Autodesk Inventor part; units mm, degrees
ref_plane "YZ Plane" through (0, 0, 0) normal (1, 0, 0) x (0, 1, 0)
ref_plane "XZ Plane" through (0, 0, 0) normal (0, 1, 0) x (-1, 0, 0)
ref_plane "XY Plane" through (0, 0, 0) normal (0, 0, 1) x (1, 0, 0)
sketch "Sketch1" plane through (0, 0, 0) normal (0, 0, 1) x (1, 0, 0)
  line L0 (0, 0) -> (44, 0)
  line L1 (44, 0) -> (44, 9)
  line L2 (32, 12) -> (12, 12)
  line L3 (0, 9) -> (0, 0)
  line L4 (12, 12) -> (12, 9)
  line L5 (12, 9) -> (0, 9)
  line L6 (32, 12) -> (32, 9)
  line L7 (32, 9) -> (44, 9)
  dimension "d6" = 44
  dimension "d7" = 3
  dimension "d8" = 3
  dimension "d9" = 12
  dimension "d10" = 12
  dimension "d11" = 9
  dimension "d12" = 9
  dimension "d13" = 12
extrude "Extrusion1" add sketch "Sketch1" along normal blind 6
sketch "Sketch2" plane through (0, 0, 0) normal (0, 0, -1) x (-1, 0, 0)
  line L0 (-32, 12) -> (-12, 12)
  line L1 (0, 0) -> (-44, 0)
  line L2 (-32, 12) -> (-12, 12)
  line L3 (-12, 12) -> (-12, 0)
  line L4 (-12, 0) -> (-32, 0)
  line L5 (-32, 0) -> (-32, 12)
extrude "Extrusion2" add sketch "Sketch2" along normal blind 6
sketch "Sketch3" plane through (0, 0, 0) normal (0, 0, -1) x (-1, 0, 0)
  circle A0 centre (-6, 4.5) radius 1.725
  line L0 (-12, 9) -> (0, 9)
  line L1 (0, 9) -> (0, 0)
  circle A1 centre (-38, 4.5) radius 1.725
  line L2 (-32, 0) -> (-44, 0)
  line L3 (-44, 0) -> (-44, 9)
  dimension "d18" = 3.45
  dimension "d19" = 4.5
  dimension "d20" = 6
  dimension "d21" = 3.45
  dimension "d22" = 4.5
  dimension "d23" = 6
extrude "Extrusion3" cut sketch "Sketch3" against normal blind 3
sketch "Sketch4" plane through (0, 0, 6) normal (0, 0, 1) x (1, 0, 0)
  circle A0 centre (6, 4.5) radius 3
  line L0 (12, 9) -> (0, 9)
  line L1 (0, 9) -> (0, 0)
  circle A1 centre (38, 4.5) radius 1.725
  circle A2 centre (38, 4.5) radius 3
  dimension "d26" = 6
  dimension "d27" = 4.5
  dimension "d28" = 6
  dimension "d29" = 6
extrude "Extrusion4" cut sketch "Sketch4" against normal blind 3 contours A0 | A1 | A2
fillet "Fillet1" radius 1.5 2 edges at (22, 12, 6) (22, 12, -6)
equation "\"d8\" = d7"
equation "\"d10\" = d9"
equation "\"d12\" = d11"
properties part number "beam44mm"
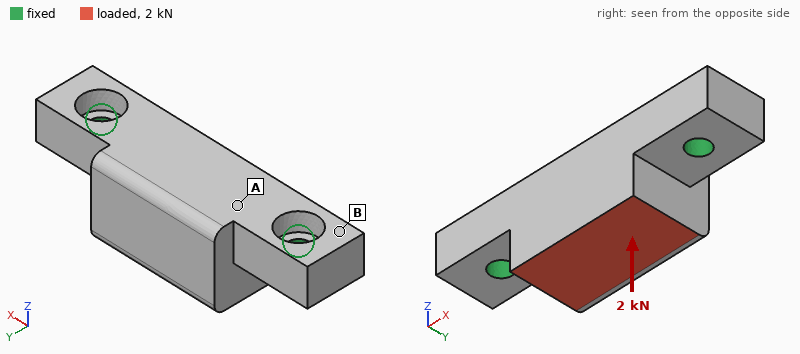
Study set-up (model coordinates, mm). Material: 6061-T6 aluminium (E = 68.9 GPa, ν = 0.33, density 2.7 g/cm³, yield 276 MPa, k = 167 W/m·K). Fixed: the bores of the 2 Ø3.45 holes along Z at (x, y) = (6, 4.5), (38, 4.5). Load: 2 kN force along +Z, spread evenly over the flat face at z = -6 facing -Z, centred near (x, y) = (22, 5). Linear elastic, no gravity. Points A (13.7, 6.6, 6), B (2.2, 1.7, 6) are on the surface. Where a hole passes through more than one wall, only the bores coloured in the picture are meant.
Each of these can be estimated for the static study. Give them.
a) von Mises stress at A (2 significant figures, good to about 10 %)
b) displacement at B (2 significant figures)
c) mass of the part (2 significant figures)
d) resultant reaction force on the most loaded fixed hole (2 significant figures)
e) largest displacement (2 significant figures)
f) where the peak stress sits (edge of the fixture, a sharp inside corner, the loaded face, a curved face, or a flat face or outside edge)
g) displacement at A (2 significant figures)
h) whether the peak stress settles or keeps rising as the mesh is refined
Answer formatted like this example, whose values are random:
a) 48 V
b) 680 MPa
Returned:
a) 51 MPa
b) 5.2 µm
c) 11 g
d) 1.0 kN
e) 26 µm
f) edge of the fixture
g) 17 µm
h) keeps rising
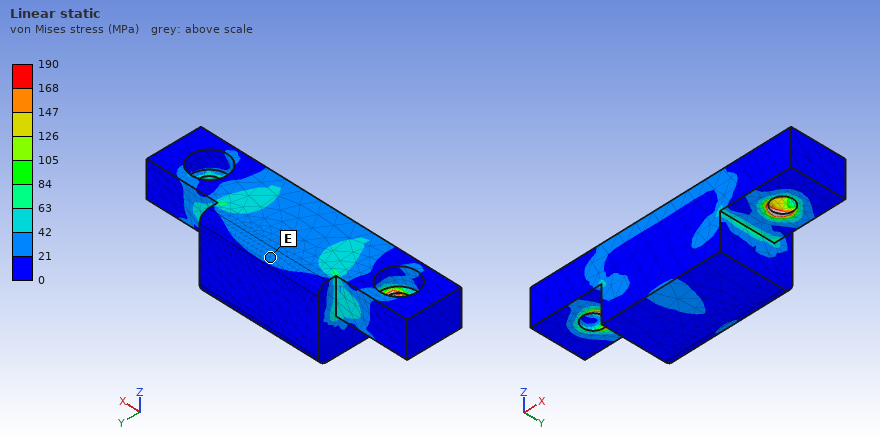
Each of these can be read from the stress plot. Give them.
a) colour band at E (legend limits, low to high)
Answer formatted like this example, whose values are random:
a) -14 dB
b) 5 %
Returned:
a) 21 to 42 MPa
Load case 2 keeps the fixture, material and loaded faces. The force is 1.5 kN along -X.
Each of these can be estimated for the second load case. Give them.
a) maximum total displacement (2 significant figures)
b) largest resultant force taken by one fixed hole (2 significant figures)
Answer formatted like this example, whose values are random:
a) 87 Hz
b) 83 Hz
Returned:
a) 12 µm
b) 870 N
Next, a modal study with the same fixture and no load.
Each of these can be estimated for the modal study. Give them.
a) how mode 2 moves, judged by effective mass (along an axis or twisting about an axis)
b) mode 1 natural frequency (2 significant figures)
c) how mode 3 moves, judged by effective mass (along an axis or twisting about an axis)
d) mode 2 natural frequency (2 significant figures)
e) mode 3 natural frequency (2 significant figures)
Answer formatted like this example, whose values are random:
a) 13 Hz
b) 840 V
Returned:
a) along Z
b) 13 kHz
c) along Y
d) 19 kHz
e) 23 kHz
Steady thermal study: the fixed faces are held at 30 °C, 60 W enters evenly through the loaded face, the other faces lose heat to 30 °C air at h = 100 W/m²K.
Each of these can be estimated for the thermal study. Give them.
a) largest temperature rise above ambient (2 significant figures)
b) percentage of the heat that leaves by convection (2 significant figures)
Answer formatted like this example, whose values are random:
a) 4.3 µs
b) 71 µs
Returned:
a) 44 K
b) 6.2 %
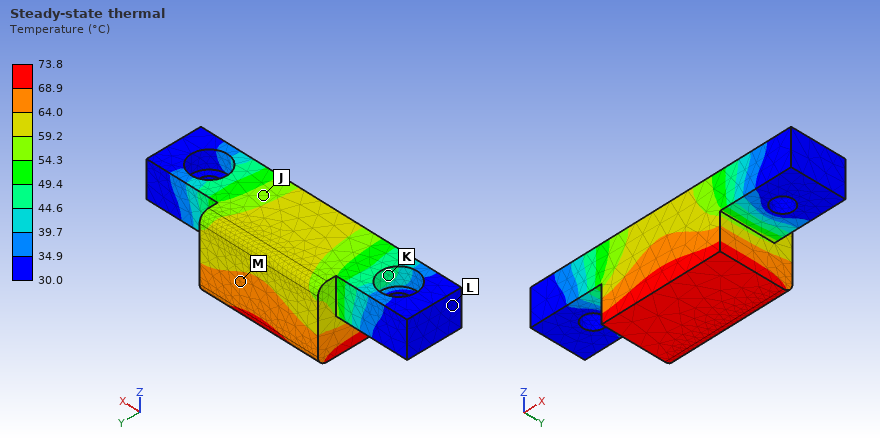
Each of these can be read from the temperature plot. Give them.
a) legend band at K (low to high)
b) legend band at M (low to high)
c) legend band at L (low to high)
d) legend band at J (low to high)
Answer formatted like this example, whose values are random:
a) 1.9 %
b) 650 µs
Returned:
a) 44.6 to 49.4 °C
b) 64.0 to 68.9 °C
c) 30.0 to 34.9 °C
d) 54.3 to 59.2 °C
